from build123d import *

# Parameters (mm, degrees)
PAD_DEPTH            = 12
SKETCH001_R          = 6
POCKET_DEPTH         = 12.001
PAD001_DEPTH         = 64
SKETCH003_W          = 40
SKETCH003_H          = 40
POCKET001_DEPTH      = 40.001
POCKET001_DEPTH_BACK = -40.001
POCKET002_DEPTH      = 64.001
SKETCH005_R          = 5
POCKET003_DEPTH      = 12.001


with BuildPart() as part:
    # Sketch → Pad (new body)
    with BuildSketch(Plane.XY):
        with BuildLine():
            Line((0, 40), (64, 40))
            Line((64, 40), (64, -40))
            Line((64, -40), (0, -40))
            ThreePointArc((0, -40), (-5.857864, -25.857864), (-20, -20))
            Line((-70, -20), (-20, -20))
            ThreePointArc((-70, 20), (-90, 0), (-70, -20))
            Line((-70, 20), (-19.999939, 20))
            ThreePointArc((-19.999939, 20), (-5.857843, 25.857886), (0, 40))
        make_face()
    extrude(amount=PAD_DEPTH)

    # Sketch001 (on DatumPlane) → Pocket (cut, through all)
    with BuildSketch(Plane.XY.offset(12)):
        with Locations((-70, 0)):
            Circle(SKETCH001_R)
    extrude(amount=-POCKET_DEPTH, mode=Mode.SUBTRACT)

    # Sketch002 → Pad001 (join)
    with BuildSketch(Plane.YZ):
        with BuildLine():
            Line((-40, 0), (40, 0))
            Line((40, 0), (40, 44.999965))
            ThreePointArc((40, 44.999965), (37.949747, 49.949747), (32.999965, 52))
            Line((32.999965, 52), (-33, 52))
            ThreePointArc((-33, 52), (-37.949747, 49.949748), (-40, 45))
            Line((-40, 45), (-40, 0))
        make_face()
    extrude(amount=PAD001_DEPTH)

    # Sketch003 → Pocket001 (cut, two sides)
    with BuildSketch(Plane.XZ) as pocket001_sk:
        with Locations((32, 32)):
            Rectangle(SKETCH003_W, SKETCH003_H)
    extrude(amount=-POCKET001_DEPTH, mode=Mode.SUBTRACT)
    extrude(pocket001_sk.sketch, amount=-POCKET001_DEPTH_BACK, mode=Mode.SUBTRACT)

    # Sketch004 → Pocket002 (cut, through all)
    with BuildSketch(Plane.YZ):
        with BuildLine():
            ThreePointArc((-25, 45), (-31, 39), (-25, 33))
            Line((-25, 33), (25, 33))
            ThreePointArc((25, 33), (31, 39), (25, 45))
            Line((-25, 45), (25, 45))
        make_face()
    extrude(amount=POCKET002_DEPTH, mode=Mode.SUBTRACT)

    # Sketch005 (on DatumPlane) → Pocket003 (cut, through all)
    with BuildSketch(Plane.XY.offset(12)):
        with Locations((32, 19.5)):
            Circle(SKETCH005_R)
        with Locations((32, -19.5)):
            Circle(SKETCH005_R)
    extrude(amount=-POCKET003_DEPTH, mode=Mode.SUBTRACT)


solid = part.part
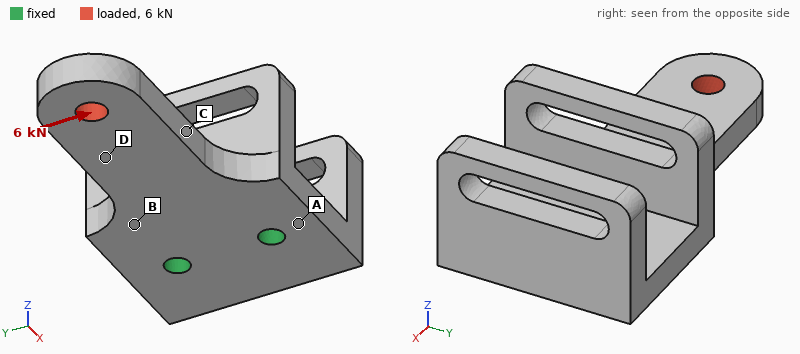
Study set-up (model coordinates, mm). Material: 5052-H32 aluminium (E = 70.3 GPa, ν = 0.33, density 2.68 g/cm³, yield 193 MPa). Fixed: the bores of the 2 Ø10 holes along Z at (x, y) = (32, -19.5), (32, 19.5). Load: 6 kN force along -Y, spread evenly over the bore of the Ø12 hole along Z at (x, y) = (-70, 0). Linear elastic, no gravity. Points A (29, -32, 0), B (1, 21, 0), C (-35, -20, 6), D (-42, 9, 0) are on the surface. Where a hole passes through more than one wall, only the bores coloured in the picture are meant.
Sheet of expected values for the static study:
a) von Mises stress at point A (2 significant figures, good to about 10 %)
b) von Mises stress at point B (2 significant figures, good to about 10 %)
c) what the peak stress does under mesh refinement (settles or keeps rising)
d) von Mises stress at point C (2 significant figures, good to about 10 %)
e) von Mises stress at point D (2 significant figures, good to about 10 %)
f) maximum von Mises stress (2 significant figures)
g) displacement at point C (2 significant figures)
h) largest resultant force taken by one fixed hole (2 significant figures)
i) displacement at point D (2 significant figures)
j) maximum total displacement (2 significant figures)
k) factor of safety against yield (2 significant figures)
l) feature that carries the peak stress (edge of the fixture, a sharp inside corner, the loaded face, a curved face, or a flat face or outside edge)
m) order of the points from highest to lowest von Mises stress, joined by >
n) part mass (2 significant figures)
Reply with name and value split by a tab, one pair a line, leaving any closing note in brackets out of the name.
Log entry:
von Mises stress at point A	20 MPa
von Mises stress at point B	53 MPa
what the peak stress does under mesh refinement	settles
von Mises stress at point C	66 MPa
von Mises stress at point D	35 MPa
maximum von Mises stress	130 MPa
displacement at point C	0.11 mm
largest resultant force taken by one fixed hole	14 kN
displacement at point D	0.12 mm
maximum total displacement	0.31 mm
factor of safety against yield	1.5
feature that carries the peak stress	a curved face
order of the points from highest to lowest von Mises stress, joined by >	C > B > D > A
part mass	430 g
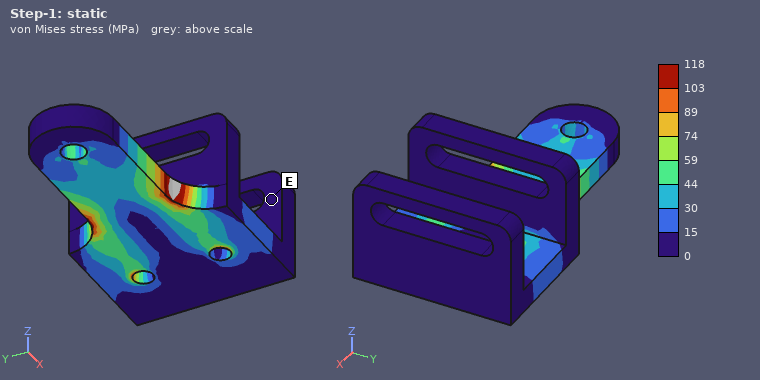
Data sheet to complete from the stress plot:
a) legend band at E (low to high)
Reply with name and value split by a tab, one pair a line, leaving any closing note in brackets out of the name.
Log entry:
legend band at E	0 to 15 MPa
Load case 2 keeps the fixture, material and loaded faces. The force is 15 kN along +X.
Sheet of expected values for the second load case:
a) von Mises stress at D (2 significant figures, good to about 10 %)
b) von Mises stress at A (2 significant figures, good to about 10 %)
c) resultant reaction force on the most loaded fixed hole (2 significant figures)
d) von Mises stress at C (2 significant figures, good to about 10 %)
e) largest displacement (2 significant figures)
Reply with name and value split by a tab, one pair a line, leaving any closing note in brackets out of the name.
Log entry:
von Mises stress at D	32 MPa
von Mises stress at A	7.7 MPa
resultant reaction force on the most loaded fixed hole	7.7 kN
von Mises stress at C	31 MPa
largest displacement	53 µm
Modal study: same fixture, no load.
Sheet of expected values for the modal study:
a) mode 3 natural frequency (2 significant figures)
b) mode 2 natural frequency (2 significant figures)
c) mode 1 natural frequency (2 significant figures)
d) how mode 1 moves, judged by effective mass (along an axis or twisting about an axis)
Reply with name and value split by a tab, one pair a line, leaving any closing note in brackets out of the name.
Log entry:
mode 3 natural frequency	3200 Hz
mode 2 natural frequency	2800 Hz
mode 1 natural frequency	940 Hz
how mode 1 moves, judged by effective mass	along Z
